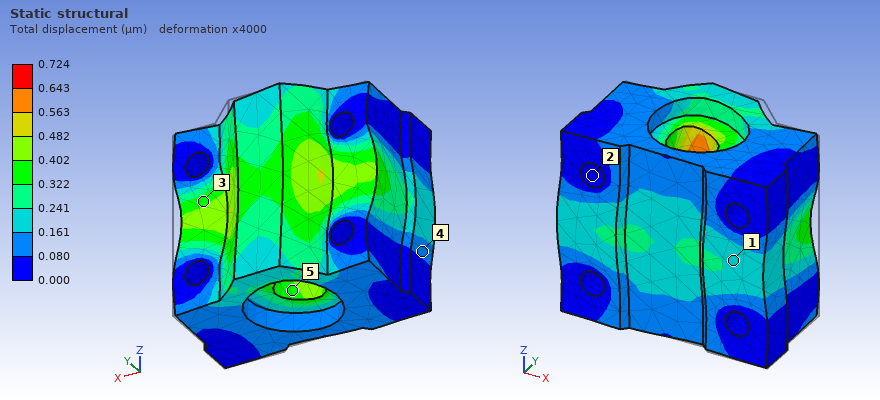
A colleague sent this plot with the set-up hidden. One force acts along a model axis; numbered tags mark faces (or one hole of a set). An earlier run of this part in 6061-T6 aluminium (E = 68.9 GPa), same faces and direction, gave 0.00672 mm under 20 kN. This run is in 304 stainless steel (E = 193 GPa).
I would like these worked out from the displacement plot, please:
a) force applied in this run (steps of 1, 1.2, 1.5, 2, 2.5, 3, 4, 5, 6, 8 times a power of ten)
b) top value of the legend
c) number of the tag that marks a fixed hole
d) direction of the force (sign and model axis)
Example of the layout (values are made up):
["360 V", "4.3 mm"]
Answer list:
["6 kN", "0.724 µm", "2", "-X"]
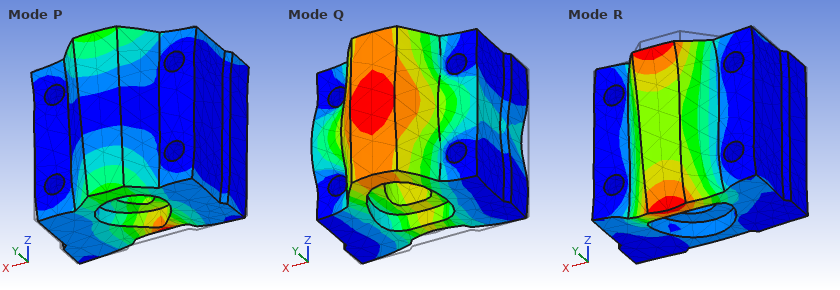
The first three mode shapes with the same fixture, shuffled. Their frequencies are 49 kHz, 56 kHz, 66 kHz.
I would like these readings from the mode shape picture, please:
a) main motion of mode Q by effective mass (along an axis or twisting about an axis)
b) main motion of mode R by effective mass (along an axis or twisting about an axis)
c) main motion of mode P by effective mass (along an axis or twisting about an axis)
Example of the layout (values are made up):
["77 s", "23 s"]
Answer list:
["along Y", "along Z", "along Z"]
